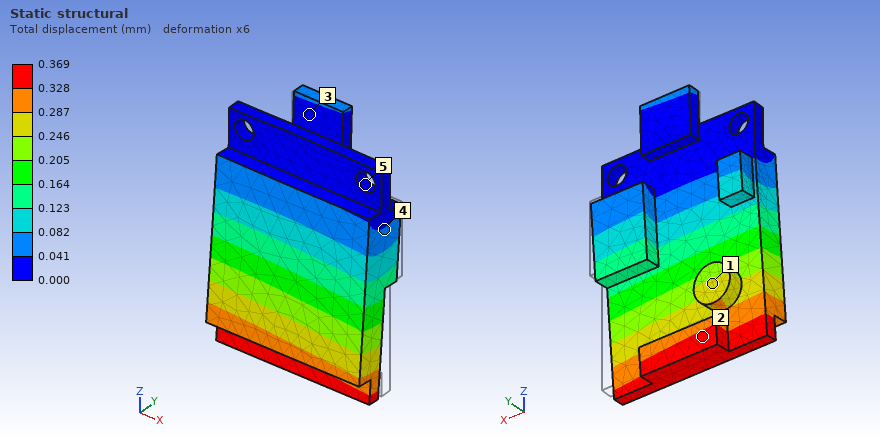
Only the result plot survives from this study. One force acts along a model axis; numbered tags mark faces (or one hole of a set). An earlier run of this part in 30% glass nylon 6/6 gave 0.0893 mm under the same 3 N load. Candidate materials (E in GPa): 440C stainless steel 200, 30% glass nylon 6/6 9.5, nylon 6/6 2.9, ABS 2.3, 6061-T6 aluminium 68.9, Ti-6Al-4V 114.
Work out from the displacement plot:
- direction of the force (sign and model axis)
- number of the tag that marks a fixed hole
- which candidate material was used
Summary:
-Y
5
ABS
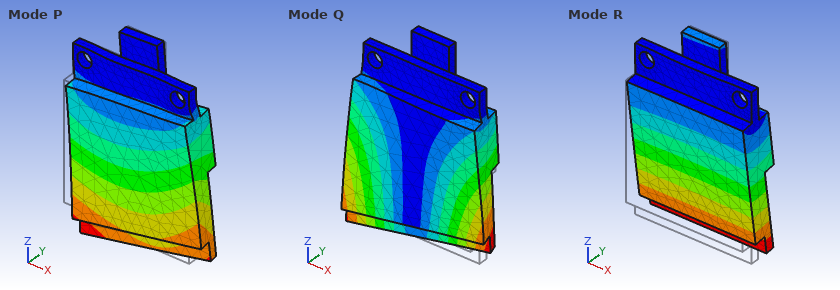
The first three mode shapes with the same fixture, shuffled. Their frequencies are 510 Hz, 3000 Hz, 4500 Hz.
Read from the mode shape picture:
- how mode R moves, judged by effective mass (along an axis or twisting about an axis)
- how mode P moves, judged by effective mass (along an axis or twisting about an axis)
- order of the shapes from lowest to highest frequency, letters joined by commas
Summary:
along Y
along X
R, Q, P
